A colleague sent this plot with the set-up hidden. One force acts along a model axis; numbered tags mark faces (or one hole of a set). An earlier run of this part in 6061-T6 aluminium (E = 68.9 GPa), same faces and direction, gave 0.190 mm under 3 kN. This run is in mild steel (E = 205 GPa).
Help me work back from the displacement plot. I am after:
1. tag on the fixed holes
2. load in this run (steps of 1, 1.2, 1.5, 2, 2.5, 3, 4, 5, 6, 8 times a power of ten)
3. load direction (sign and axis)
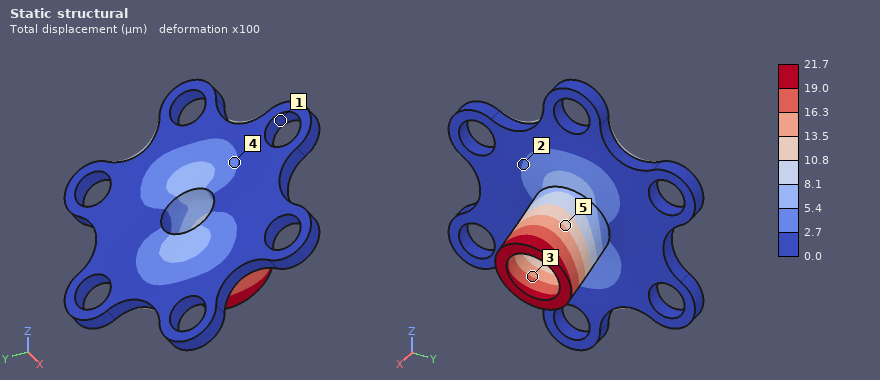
1
1 kN
-Z
